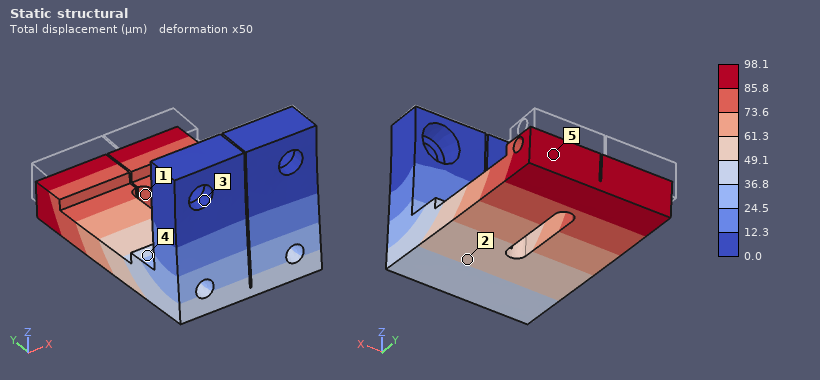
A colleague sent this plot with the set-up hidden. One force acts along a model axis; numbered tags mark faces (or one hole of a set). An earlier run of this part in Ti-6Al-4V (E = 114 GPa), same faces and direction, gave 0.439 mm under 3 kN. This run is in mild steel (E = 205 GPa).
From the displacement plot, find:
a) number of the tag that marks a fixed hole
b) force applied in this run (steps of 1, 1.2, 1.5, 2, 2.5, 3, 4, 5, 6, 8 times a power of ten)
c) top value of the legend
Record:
3
1.2 kN
98.1 µm
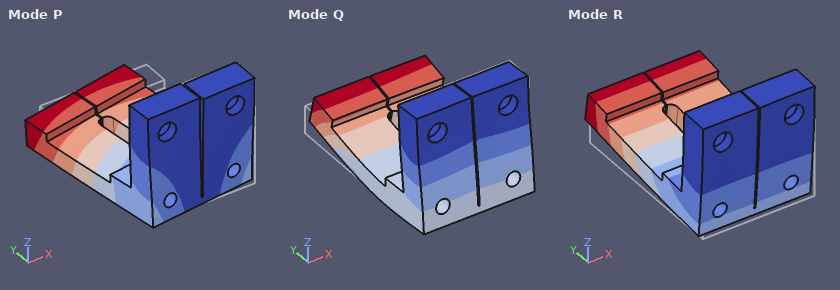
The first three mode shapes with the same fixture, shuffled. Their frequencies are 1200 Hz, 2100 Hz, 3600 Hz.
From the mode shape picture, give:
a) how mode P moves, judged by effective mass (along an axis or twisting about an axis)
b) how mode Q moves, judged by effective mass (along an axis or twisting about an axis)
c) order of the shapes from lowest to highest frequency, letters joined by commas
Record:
along X
along Y
R, P, Q
